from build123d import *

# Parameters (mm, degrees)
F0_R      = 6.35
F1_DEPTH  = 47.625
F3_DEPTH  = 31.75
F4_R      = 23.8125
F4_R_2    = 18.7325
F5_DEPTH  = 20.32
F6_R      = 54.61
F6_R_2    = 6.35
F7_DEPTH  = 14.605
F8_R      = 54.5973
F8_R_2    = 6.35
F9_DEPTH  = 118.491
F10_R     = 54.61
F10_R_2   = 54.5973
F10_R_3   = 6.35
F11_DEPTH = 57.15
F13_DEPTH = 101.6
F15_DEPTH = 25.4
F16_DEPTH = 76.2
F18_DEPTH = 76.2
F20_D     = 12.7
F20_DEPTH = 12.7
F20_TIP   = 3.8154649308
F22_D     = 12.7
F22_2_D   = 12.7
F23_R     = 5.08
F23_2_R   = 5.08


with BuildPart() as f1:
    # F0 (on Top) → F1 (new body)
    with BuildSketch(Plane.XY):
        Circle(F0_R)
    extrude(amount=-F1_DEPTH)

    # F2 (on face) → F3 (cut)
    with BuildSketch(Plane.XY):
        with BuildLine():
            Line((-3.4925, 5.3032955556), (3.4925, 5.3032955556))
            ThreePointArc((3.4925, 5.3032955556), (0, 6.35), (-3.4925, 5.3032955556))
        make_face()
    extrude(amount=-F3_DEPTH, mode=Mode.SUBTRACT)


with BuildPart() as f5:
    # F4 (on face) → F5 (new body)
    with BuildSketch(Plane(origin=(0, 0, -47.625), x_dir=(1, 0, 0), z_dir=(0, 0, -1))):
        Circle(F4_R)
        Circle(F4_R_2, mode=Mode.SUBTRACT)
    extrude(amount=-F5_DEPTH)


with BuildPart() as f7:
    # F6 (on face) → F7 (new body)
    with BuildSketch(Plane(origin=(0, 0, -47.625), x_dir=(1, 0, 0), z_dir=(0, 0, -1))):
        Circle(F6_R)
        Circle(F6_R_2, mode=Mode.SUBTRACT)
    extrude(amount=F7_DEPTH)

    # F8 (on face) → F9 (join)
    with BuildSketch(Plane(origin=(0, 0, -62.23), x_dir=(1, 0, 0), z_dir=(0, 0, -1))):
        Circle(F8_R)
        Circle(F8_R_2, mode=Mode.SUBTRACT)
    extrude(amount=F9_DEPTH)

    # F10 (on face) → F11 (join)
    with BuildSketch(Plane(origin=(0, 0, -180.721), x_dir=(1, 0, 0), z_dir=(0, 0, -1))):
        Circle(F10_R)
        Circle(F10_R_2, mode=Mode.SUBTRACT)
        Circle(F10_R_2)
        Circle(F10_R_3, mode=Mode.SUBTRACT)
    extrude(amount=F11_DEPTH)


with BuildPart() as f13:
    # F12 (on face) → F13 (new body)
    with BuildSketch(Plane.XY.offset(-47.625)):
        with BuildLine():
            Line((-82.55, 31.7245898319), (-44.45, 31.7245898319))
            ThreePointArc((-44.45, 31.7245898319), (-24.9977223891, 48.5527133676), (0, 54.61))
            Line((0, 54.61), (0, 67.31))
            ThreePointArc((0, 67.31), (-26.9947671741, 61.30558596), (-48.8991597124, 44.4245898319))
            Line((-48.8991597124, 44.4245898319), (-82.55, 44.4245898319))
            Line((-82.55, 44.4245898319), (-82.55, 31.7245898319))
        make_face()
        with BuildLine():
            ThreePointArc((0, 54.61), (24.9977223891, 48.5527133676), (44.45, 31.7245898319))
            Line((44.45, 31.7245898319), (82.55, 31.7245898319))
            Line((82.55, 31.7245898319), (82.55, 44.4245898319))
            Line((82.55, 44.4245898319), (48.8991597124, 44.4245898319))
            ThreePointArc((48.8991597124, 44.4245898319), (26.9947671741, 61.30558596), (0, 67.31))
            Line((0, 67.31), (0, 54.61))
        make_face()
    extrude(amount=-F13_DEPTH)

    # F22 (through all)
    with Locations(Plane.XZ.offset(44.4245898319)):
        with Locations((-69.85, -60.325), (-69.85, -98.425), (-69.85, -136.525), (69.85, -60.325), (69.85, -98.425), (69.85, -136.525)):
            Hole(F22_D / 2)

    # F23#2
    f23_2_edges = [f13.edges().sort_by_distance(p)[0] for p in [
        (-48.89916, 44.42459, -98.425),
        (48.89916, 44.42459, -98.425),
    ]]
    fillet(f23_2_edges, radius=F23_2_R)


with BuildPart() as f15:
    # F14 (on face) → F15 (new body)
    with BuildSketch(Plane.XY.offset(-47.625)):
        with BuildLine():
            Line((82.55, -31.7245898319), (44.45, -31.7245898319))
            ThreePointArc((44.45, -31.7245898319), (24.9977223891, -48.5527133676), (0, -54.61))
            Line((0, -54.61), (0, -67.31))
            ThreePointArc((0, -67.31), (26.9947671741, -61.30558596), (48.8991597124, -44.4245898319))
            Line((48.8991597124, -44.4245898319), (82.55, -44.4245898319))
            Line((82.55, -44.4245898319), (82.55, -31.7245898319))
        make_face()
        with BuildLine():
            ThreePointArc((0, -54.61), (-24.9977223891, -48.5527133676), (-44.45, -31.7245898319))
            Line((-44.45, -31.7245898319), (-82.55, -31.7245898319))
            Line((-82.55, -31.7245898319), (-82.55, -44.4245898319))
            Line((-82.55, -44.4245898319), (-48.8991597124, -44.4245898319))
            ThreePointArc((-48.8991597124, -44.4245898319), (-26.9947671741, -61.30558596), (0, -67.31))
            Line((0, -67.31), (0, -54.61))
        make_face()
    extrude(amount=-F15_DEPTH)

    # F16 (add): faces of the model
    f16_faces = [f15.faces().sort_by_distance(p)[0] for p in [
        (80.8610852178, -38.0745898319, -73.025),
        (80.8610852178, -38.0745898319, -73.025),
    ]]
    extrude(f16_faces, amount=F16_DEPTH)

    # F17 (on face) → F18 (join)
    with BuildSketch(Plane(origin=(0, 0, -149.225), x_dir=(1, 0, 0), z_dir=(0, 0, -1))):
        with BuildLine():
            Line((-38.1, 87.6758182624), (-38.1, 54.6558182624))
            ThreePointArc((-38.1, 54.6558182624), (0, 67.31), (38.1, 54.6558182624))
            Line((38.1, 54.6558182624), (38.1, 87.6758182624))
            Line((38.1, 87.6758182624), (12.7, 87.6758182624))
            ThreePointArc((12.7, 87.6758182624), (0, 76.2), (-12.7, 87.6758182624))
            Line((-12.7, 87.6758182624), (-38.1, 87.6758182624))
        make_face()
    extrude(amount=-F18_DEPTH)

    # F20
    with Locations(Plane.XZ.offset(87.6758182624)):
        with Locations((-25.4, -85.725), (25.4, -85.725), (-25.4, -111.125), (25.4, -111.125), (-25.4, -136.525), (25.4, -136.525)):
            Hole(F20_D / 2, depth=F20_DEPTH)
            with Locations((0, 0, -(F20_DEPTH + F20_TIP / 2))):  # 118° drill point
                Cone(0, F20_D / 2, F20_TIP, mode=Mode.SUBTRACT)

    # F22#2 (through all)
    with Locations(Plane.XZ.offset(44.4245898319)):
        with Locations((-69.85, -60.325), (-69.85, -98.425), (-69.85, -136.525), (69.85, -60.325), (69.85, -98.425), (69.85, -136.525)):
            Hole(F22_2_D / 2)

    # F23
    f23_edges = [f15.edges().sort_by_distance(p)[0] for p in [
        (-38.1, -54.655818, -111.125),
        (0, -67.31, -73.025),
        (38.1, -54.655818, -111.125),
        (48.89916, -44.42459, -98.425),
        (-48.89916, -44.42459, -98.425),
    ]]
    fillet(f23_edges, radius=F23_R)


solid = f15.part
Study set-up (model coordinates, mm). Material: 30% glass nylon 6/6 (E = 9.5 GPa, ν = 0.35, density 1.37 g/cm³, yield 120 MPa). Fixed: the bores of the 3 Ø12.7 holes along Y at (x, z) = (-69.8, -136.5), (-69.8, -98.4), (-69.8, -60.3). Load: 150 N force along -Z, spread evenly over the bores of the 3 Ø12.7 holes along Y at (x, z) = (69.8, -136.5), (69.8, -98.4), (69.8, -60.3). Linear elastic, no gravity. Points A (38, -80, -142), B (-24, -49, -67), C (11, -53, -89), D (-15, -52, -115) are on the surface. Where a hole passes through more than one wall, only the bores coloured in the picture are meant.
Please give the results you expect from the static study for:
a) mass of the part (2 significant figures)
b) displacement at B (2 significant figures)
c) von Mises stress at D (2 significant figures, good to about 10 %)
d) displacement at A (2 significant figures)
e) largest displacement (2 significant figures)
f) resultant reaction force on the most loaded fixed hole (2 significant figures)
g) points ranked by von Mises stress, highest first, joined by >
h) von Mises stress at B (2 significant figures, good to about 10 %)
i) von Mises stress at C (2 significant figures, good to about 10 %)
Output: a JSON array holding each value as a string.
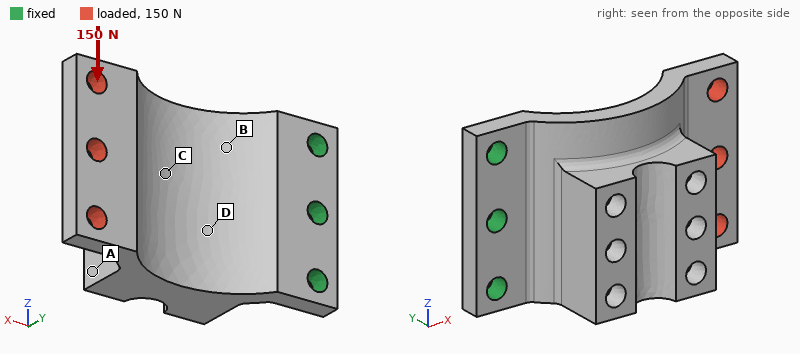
["450 g", "16 µm", "1.2 MPa", "38 µm", "75 µm", "270 N", "B > D > C > A", "1.9 MPa", "0.60 MPa"]
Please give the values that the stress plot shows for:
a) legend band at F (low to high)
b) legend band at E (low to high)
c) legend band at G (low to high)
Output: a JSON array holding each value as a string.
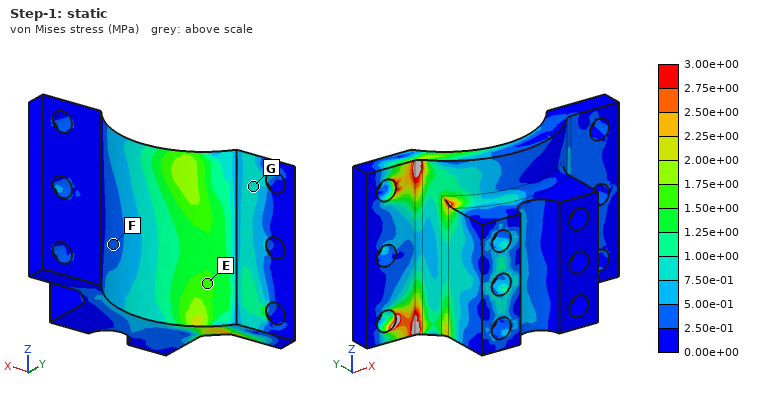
["2.50e-01 to 5.00e-01 MPa", "1.50e+00 to 1.75e+00 MPa", "7.50e-01 to 1.00e+00 MPa"]
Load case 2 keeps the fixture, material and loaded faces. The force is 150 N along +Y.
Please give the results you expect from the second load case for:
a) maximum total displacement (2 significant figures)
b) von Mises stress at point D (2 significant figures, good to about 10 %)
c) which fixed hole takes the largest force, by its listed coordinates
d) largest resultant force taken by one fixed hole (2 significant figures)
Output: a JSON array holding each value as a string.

["0.72 mm", "1.7 MPa", "(-69.8, -98.4)", "81 N"]
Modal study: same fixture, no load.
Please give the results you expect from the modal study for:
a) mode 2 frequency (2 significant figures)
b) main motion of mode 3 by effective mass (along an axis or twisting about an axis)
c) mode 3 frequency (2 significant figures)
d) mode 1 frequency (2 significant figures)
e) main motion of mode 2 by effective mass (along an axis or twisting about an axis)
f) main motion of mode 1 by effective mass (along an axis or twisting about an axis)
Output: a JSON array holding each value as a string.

["730 Hz", "along Z", "1300 Hz", "220 Hz", "along Z", "along Y"]
